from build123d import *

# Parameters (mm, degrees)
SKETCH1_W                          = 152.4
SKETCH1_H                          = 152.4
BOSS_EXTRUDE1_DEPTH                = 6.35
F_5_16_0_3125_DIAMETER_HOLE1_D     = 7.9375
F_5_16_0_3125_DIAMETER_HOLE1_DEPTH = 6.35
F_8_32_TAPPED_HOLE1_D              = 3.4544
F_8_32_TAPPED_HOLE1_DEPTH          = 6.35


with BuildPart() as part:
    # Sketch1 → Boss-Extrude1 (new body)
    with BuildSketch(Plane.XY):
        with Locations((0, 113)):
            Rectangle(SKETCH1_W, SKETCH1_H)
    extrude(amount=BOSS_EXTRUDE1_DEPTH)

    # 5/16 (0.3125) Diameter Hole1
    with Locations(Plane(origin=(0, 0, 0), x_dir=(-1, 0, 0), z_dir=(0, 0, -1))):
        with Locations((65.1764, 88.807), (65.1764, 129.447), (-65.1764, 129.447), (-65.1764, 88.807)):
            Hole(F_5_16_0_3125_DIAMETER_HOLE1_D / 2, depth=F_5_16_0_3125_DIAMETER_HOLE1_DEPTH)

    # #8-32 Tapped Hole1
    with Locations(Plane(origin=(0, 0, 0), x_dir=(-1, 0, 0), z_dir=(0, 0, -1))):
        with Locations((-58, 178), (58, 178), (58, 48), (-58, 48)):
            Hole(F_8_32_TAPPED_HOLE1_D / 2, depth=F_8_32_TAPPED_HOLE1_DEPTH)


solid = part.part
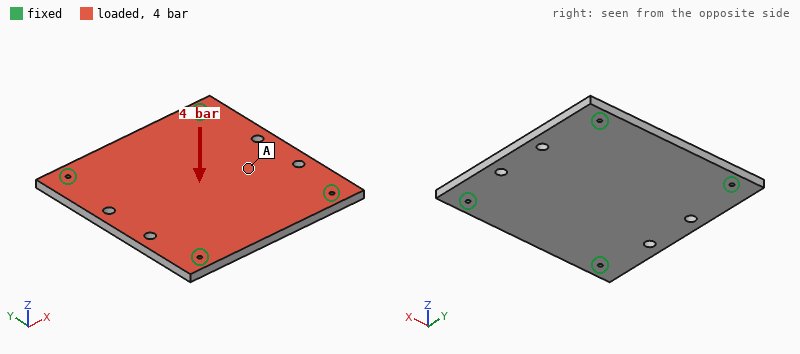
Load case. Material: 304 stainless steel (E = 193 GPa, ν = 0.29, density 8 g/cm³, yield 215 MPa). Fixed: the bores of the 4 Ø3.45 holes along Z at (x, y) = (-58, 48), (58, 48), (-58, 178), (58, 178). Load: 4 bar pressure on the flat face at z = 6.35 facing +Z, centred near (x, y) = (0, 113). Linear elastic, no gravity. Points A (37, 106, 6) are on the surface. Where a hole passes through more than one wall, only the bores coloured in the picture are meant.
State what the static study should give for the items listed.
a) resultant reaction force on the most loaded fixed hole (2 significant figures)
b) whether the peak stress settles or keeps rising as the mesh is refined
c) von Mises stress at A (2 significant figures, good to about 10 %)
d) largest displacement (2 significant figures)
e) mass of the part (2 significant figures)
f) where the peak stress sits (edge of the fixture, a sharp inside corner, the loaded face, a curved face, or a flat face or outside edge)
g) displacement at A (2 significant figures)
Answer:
2.3 kN
keeps rising
52 MPa
0.19 mm
1.2 kg
edge of the fixture
0.16 mm
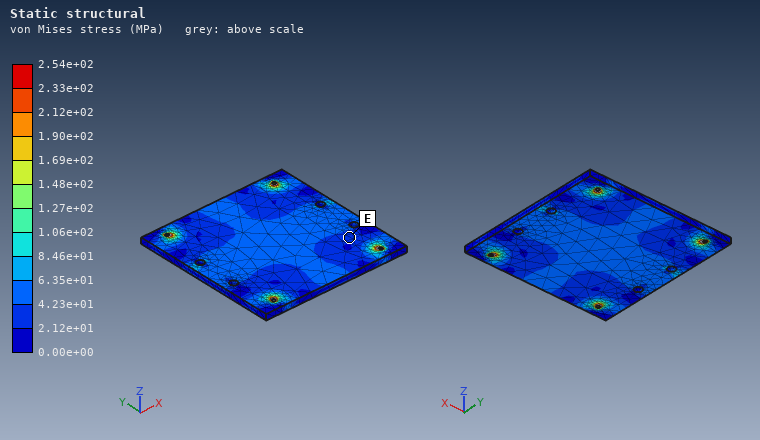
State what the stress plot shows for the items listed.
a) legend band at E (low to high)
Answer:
2.12e+01 to 4.23e+01 MPa
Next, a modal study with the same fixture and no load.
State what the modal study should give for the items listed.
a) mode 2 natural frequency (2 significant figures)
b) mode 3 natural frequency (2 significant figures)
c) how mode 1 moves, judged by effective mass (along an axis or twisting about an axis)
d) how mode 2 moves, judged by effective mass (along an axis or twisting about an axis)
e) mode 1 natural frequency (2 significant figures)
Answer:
1900 Hz
2200 Hz
along Z
twisting about Y
1200 Hz
